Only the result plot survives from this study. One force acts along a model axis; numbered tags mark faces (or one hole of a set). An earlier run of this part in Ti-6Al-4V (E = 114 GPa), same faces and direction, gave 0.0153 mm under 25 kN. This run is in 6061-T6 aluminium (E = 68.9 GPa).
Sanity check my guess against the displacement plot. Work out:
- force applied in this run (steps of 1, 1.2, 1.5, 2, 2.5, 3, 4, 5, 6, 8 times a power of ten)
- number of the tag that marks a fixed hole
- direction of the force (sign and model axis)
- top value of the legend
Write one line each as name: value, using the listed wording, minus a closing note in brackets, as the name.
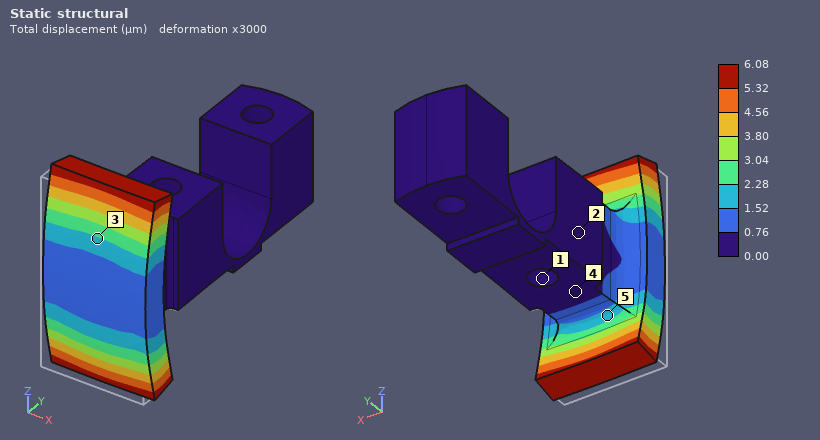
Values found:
force applied in this run: 6 kN
number of the tag that marks a fixed hole: 1
direction of the force: +Y
top value of the legend: 6.08 µm
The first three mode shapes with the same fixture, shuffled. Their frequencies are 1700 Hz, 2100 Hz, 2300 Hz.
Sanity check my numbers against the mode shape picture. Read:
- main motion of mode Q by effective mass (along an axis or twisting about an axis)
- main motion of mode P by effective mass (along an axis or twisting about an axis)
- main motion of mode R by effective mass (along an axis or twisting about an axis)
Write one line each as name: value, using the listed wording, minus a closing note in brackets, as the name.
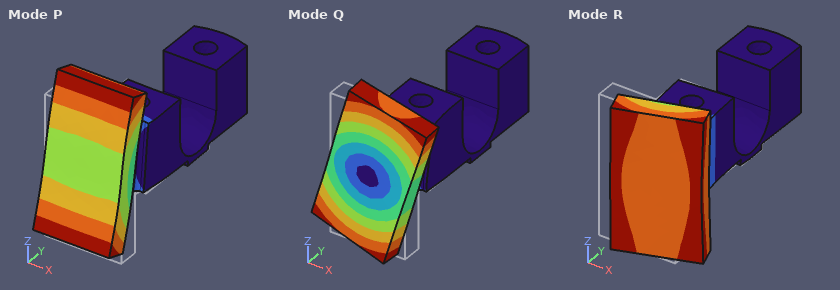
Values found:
main motion of mode Q by effective mass: twisting about Y
main motion of mode P by effective mass: along Z
main motion of mode R by effective mass: along X
